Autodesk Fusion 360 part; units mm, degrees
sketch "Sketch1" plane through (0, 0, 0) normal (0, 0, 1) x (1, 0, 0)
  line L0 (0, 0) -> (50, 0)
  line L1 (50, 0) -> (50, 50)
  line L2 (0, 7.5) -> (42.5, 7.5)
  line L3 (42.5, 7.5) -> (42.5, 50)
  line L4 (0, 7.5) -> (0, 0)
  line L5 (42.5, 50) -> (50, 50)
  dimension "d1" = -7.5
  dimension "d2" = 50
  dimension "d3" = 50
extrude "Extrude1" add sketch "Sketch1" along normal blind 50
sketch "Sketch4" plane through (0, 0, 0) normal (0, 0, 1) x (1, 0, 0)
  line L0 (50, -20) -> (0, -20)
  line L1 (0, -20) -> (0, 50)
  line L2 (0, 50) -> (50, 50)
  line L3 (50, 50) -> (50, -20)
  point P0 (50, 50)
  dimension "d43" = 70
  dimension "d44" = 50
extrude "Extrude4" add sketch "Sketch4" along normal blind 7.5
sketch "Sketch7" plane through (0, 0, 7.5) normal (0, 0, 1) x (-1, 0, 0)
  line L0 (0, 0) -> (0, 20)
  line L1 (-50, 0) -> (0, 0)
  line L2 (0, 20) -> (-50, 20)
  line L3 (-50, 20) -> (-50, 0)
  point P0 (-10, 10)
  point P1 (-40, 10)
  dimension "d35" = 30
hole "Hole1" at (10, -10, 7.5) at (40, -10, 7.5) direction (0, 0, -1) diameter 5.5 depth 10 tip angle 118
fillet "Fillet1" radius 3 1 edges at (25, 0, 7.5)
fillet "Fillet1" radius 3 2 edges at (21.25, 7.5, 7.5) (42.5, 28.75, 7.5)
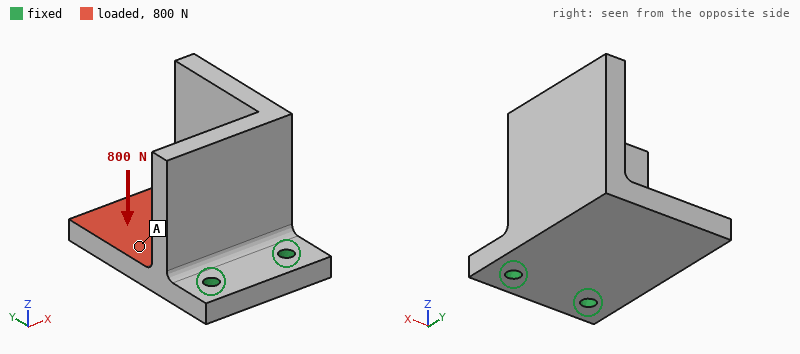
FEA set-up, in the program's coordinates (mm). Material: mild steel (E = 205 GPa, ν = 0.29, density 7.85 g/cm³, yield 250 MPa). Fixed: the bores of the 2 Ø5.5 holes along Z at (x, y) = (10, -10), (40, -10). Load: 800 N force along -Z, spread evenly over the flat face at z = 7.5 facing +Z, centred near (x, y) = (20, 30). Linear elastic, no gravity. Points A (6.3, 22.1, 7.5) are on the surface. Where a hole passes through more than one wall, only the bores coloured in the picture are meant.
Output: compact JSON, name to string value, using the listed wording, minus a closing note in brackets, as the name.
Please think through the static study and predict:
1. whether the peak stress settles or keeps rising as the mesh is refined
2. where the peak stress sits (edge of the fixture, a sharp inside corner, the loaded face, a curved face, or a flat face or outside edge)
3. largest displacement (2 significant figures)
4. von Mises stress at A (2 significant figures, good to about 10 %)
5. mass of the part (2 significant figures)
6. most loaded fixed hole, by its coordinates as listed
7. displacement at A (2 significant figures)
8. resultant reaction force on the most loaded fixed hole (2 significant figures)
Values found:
{"whether the peak stress settles or keeps rising as the mesh is refined": "keeps rising", "where the peak stress sits": "edge of the fixture", "largest displacement": "74 µm", "von Mises stress at A": "11 MPa", "mass of the part": "440 g", "most loaded fixed hole, by its coordinates as listed": "(10, -10)", "displacement at A": "30 µm", "resultant reaction force on the most loaded fixed hole": "520 N"}
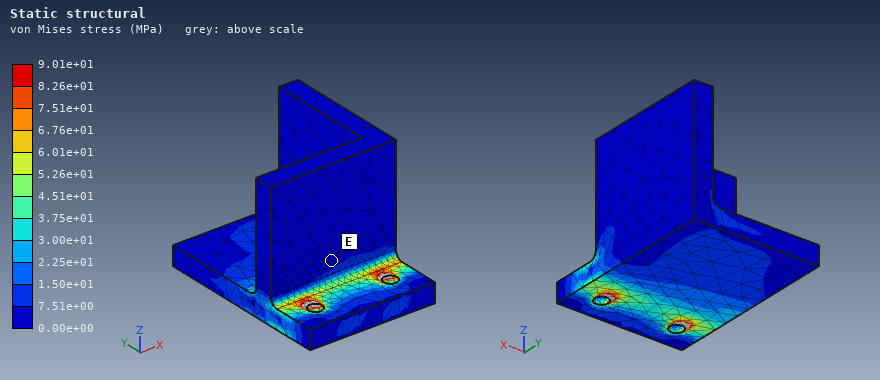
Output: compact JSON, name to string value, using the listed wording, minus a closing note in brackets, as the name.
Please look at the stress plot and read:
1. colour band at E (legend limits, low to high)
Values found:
{"colour band at E": "0.00e+00 to 7.51e+00 MPa"}
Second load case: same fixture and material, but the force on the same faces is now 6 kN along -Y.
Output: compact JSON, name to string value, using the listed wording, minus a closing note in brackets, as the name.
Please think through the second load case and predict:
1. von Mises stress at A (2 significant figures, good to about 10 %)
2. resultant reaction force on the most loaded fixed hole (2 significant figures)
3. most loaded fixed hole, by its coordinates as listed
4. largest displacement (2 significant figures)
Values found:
{"von Mises stress at A": "39 MPa", "resultant reaction force on the most loaded fixed hole": "4.0 kN", "most loaded fixed hole, by its coordinates as listed": "(10, -10)", "largest displacement": "67 µm"}
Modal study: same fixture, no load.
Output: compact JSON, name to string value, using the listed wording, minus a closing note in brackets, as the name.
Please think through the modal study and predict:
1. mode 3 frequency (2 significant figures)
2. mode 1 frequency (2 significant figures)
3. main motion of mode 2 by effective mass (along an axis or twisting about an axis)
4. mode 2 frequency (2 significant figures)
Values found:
{"mode 3 frequency": "4400 Hz", "mode 1 frequency": "1100 Hz", "main motion of mode 2 by effective mass": "along X", "mode 2 frequency": "3100 Hz"}
